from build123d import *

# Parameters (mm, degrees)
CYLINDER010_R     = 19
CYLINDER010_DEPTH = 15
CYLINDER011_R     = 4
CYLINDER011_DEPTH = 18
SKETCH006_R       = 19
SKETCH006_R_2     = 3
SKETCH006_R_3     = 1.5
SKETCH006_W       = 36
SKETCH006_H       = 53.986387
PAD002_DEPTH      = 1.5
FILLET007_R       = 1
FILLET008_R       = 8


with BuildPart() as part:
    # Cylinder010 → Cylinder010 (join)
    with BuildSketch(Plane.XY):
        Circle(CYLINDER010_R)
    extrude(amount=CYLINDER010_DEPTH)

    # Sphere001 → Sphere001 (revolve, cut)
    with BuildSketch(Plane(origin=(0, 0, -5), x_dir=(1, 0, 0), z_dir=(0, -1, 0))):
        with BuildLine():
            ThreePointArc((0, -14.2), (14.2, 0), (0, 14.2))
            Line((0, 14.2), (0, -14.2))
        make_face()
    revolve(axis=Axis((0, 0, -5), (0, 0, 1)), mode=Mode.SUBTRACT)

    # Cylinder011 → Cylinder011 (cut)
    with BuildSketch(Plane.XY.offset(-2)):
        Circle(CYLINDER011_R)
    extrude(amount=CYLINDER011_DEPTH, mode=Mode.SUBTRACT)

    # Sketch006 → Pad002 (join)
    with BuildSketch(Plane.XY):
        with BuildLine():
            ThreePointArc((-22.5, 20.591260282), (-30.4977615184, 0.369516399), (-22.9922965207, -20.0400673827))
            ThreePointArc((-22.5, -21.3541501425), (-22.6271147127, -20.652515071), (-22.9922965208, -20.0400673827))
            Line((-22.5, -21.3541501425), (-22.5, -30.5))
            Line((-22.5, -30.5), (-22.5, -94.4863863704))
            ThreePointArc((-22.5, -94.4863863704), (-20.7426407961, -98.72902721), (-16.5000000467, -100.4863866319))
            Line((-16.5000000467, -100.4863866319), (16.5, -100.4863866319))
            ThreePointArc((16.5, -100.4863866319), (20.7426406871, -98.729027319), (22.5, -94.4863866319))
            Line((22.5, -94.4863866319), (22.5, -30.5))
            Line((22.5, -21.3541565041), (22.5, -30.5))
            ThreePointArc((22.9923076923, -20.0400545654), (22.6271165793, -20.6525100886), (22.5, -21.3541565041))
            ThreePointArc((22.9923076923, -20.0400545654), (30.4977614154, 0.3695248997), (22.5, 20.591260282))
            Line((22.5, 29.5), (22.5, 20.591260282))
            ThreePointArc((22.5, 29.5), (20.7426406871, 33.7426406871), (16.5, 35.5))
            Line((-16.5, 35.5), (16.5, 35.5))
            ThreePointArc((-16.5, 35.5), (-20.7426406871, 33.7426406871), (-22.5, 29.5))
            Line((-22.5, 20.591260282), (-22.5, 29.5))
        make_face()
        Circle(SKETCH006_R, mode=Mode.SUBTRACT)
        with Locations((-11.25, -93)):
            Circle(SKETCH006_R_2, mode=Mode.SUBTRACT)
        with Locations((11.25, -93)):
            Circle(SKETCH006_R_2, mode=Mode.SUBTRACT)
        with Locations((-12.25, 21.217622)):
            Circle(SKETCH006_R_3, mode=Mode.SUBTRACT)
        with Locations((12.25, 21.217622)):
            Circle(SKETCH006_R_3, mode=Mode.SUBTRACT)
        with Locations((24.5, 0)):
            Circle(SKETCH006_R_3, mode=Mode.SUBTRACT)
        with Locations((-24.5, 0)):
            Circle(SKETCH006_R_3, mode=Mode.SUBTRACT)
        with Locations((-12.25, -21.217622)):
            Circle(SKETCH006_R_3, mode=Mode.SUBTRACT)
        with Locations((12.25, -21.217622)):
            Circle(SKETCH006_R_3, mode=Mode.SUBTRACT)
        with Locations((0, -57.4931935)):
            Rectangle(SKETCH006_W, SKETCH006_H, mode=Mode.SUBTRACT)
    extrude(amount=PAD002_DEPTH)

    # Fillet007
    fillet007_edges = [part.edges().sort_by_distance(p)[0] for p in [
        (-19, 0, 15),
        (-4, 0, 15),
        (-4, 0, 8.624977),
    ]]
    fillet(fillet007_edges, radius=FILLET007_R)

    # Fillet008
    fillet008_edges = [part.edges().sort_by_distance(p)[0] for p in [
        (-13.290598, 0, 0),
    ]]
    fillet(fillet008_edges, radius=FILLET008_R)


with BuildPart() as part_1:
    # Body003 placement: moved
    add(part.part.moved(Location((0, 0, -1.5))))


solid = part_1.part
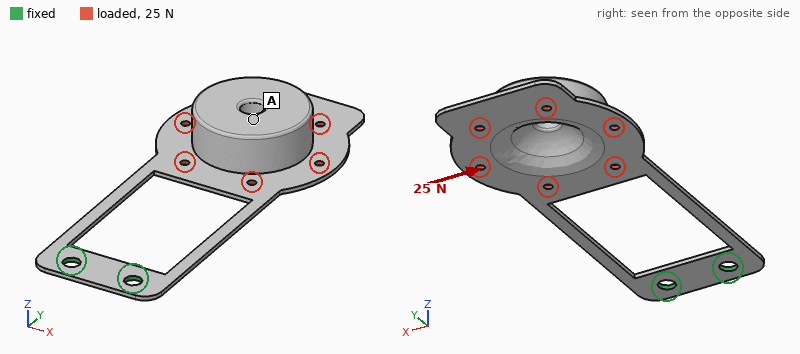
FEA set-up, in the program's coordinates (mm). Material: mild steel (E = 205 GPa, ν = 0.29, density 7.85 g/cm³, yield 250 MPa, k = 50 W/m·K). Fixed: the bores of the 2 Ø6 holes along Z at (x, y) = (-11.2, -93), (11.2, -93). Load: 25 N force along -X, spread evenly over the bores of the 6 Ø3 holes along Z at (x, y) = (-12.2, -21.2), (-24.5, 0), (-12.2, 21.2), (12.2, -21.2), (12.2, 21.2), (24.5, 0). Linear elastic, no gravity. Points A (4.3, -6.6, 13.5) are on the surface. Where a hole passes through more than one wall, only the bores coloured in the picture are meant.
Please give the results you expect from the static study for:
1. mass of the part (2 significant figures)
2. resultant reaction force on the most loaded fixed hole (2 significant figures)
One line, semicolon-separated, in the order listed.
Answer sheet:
150 g; 61 N
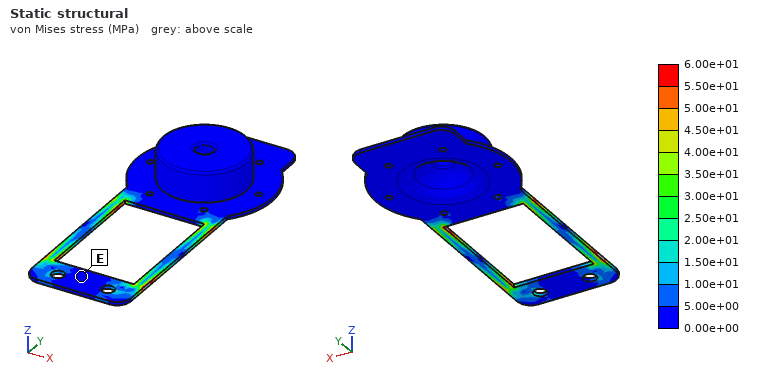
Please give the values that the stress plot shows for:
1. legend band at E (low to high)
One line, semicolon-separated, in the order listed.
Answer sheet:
0.00e+00 to 5.00e+00 MPa
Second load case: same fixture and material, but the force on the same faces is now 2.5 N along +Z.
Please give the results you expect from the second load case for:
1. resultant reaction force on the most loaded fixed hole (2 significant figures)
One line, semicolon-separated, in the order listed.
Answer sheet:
1.3 N
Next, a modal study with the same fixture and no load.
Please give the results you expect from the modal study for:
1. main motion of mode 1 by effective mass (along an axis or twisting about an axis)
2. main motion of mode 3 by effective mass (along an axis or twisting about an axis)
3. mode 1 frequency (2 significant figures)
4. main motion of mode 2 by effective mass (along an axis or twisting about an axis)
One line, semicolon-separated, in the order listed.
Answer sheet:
along Z; along X; 20 Hz; along X
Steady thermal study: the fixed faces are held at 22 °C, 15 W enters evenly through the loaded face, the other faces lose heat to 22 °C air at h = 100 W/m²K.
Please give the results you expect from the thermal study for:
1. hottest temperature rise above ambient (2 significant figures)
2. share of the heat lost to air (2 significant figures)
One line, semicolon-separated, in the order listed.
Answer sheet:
28 K; 100 %
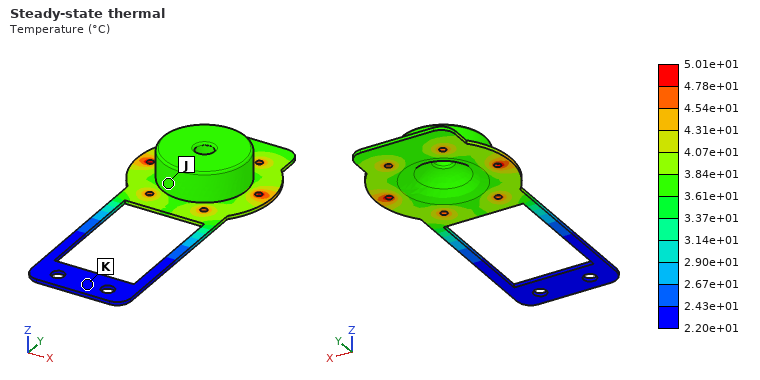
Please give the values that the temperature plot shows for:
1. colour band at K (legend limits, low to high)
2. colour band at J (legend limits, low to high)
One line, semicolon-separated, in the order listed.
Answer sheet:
2.20e+01 to 2.43e+01 °C; 3.61e+01 to 3.84e+01 °C
